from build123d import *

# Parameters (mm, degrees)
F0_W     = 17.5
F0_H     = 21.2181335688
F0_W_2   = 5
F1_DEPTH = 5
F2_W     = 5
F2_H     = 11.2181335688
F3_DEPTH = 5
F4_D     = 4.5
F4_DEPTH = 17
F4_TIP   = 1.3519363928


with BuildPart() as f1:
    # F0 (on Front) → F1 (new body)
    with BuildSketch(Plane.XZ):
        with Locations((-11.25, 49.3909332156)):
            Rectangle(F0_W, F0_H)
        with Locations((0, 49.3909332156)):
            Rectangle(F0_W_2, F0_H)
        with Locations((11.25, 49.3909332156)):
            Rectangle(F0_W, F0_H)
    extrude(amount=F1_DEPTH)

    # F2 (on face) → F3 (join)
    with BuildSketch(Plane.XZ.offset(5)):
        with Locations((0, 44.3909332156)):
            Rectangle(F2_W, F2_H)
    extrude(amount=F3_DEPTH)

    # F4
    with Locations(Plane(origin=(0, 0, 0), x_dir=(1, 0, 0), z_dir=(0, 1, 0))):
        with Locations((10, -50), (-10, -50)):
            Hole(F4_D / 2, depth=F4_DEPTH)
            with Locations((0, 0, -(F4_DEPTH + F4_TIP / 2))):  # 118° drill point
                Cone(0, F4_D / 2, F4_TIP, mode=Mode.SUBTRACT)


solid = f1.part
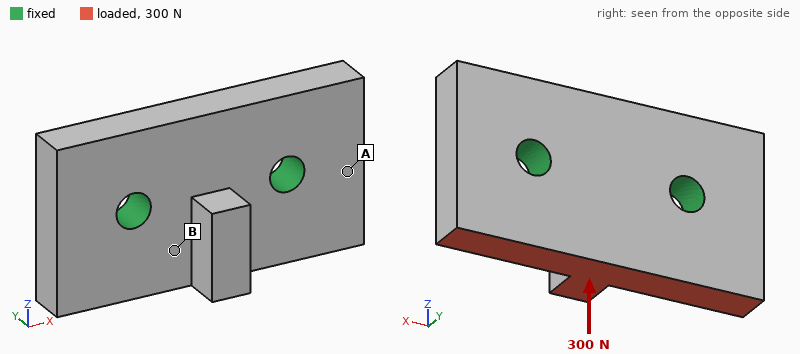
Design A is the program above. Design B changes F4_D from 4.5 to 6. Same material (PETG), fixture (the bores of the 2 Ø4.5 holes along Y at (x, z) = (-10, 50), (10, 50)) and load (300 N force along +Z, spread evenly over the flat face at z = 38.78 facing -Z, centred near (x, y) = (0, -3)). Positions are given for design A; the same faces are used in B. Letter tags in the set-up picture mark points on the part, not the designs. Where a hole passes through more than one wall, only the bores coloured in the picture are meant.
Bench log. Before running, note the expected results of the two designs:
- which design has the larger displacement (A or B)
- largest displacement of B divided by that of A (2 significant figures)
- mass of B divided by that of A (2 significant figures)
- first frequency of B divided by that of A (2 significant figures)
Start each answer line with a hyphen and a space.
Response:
- A
- 0.89
- 0.97
- 1.2
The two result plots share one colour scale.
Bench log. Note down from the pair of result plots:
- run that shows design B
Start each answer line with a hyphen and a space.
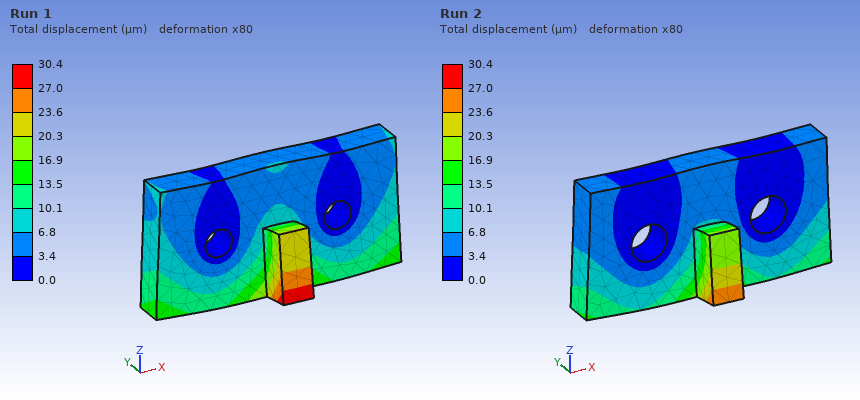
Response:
- Run 2
